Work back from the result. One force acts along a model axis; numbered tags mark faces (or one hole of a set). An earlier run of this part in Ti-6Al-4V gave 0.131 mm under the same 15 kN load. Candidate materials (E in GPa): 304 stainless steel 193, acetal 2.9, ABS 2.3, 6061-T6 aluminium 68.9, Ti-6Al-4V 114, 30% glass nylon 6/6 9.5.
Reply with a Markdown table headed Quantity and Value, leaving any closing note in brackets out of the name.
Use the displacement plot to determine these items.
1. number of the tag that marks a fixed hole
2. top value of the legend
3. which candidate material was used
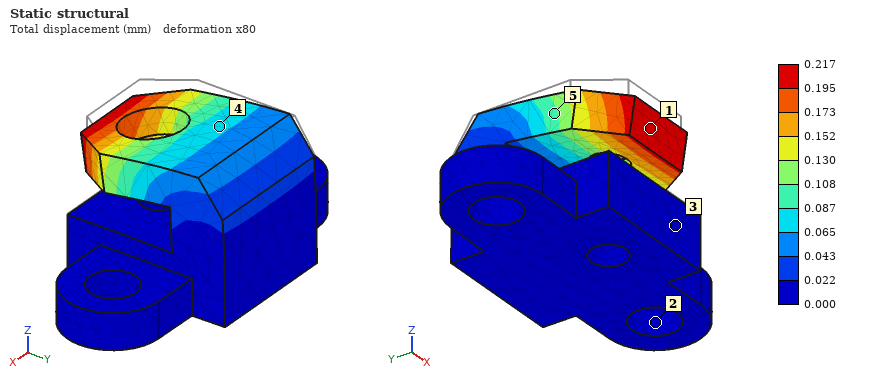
| Quantity | Value |
|---|---|
| number of the tag that marks a fixed hole | 2 |
| top value of the legend | 0.217 mm |
| which candidate material was used | 6061-T6 aluminium |
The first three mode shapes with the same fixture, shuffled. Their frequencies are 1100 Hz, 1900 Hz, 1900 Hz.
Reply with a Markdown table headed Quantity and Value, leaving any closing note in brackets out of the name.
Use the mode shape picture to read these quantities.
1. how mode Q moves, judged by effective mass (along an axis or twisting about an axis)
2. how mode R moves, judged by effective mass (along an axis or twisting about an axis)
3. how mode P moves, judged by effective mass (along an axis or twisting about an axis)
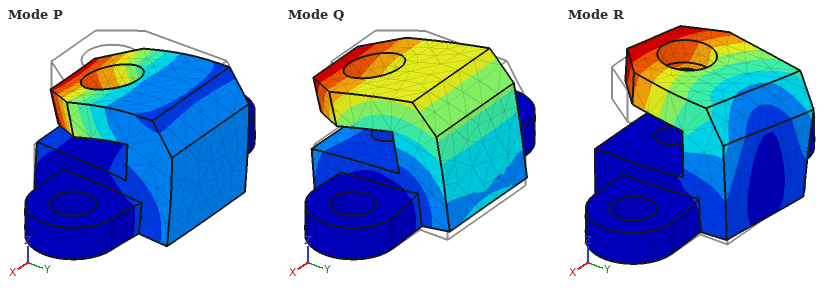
| Quantity | Value |
|---|---|
| how mode Q moves, judged by effective mass | along Y |
| how mode R moves, judged by effective mass | along X |
| how mode P moves, judged by effective mass | along Z |
